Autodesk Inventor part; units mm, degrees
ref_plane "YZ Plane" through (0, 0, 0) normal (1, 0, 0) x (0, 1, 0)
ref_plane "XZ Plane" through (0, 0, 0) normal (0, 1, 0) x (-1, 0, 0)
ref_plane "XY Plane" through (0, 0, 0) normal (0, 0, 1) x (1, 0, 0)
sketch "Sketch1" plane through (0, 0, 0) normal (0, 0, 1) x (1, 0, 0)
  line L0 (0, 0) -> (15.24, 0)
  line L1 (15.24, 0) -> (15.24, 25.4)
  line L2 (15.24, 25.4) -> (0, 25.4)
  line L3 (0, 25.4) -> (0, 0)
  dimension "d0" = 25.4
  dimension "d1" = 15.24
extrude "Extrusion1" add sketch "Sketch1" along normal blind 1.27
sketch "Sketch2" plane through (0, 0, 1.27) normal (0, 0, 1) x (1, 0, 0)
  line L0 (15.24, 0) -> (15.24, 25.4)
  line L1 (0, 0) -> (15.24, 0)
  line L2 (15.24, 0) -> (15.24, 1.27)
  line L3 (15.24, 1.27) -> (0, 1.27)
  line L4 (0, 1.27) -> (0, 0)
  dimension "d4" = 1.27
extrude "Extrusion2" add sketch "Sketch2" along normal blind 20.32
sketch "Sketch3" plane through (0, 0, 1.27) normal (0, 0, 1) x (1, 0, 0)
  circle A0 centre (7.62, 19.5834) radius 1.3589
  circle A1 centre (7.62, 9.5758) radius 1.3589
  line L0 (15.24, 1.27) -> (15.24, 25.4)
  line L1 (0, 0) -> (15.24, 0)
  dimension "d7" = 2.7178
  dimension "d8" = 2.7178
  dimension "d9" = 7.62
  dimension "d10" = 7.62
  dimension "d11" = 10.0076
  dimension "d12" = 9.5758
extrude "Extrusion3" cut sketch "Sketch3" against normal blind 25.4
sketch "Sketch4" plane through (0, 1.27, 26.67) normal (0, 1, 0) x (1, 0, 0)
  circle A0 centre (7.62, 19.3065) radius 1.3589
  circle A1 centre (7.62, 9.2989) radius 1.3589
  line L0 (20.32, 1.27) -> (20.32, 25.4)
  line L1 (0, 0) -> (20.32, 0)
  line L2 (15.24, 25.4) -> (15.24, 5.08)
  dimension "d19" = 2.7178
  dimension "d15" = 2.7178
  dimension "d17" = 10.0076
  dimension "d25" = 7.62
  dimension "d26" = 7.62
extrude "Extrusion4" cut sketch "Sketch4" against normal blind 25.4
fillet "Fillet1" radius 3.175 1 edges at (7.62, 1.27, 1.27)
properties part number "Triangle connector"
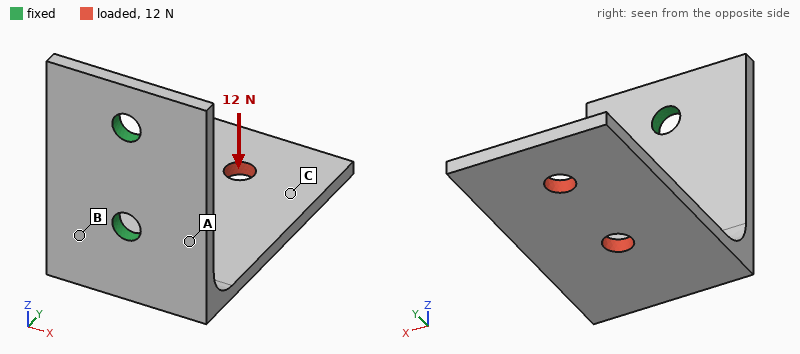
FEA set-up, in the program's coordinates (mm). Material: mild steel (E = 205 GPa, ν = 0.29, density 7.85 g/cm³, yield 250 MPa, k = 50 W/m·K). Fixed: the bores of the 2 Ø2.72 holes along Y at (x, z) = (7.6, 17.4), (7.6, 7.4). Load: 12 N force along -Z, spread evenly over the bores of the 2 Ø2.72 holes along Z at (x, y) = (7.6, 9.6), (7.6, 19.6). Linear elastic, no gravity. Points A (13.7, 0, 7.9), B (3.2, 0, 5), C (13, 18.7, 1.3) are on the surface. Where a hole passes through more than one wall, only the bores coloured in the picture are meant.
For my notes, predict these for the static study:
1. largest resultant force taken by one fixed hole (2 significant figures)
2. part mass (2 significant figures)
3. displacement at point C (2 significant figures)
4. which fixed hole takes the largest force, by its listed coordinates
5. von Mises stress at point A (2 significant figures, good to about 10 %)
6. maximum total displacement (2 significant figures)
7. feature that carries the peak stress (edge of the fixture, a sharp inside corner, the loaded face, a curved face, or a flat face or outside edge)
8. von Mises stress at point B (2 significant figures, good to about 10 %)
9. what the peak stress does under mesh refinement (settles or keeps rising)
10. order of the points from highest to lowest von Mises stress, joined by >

11 N
7.0 g
45 µm
(7.6, 7.4)
16 MPa
67 µm
edge of the fixture
32 MPa
keeps rising
B > A > C
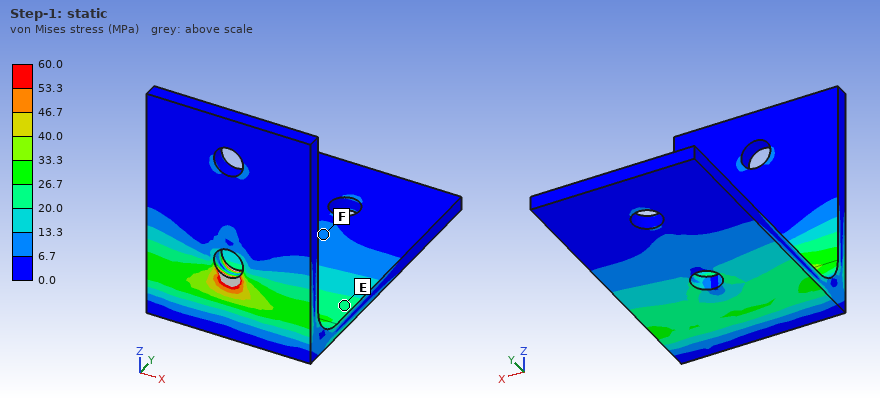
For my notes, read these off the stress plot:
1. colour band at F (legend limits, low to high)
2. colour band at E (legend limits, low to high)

6.7 to 13.3 MPa
20.0 to 26.7 MPa
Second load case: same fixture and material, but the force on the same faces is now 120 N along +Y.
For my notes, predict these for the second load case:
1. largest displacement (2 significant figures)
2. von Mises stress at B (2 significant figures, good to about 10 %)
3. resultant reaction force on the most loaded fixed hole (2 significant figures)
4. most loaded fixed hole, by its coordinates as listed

0.10 mm
91 MPa
140 N
(7.6, 7.4)
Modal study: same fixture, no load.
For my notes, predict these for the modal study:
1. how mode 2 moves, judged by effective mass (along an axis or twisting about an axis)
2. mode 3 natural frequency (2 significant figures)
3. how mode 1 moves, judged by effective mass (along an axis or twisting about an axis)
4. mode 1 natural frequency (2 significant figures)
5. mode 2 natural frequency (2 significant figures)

along X
6300 Hz
along Z
1400 Hz
2700 Hz
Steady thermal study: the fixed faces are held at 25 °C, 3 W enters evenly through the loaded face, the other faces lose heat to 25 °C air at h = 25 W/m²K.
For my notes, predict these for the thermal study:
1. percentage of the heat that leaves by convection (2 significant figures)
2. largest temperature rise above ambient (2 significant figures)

26 %
50 K
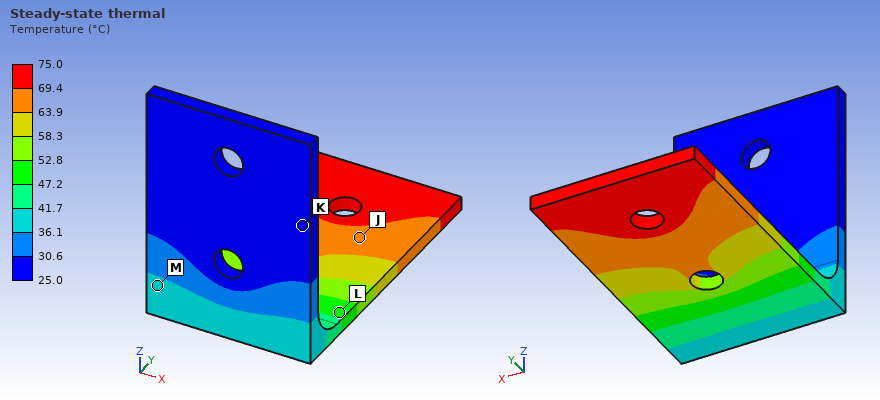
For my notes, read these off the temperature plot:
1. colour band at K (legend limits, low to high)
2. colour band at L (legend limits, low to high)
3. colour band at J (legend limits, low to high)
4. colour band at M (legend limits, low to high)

25.0 to 30.6 °C
47.2 to 52.8 °C
63.9 to 69.4 °C
36.1 to 41.7 °C
